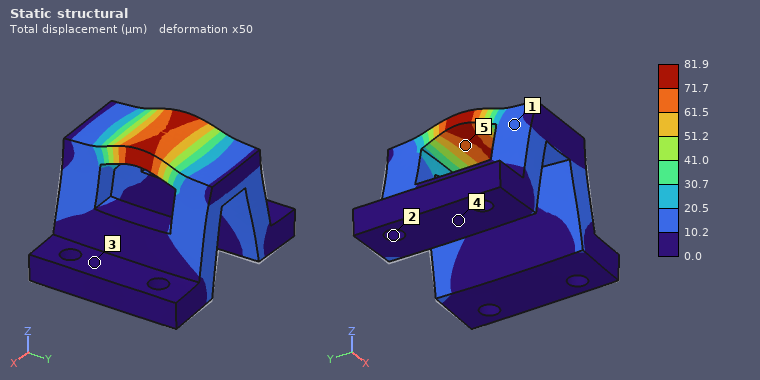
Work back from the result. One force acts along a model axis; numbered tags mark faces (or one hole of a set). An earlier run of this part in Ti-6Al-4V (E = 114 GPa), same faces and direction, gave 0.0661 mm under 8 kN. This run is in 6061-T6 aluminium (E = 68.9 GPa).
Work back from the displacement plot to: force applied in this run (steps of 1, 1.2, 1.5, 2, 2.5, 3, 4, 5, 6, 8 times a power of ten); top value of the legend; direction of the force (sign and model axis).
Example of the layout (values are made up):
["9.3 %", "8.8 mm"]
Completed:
["6 kN", "81.9 µm", "+Z"]
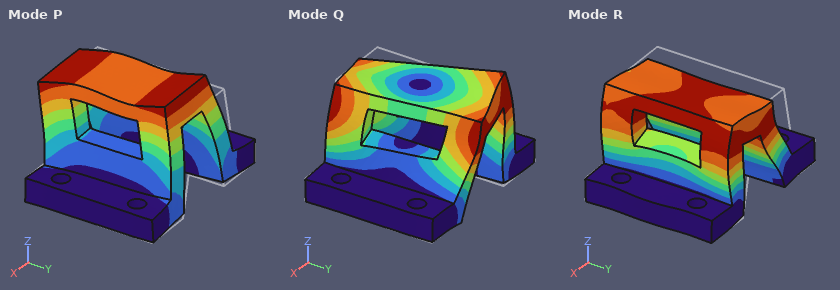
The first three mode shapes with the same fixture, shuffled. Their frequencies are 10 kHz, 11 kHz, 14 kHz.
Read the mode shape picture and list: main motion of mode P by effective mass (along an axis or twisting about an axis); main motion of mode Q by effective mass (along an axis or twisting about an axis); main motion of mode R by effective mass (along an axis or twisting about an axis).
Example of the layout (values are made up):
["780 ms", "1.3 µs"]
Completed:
["along Y", "twisting about Z", "along X"]
